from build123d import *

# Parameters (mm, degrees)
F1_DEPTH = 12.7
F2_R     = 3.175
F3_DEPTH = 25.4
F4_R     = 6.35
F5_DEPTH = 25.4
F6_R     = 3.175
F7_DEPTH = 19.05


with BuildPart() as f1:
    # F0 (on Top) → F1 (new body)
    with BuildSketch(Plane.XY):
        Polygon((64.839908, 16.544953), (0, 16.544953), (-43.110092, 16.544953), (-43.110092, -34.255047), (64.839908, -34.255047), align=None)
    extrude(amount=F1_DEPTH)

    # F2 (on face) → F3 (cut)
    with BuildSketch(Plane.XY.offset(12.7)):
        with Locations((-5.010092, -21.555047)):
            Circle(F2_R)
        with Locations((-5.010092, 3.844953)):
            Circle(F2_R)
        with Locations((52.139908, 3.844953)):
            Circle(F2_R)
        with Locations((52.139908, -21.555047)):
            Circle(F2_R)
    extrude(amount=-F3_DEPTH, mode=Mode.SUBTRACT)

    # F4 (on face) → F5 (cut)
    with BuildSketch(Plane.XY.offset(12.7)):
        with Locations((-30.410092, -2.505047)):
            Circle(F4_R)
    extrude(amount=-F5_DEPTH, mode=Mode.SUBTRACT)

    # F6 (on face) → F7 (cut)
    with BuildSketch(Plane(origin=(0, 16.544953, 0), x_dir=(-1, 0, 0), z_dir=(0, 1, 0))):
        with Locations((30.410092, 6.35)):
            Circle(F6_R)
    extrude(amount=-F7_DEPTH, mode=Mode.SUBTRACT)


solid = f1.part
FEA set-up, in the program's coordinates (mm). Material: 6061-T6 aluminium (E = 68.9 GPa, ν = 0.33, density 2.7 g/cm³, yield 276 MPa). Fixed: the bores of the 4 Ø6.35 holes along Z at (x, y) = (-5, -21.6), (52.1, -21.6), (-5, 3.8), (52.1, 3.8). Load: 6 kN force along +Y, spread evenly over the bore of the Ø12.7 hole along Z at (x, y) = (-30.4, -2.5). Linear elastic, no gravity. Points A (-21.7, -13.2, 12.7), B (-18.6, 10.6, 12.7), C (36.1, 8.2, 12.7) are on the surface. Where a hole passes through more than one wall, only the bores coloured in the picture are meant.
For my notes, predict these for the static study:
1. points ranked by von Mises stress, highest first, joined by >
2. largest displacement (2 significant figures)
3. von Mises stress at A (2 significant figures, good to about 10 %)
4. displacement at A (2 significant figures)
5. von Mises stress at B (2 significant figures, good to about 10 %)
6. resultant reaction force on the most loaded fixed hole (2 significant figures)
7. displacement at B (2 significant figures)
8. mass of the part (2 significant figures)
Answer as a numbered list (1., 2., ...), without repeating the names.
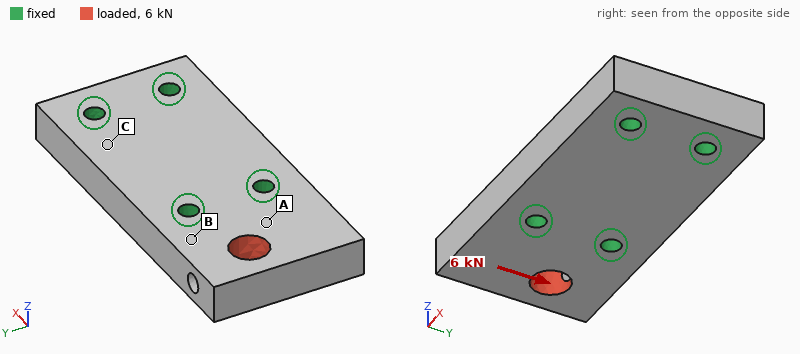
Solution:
1. A > B > C
2. 28 µm
3. 20 MPa
4. 9.5 µm
5. 12 MPa
6. 5.1 kN
7. 9.7 µm
8. 180 g
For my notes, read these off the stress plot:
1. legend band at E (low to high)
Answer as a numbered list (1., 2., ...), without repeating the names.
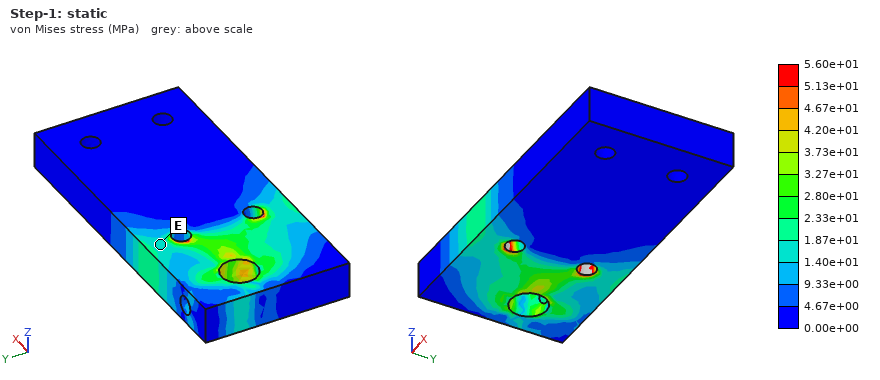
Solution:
1. 1.40e+01 to 1.87e+01 MPa
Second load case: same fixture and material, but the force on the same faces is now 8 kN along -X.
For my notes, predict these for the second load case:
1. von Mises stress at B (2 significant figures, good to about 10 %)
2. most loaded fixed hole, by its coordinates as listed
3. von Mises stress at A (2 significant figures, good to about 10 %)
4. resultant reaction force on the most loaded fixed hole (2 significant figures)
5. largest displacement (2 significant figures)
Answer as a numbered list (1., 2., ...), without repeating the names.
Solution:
1. 17 MPa
2. (-5, 3.8)
3. 20 MPa
4. 5.1 kN
5. 17 µm
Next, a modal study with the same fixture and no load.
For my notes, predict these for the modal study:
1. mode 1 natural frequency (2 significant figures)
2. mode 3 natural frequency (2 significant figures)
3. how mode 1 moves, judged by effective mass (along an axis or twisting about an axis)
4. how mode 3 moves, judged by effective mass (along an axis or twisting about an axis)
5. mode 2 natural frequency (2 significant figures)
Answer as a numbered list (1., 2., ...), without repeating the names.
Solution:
1. 6700 Hz
2. 13 kHz
3. along Z
4. along Y
5. 11 kHz
